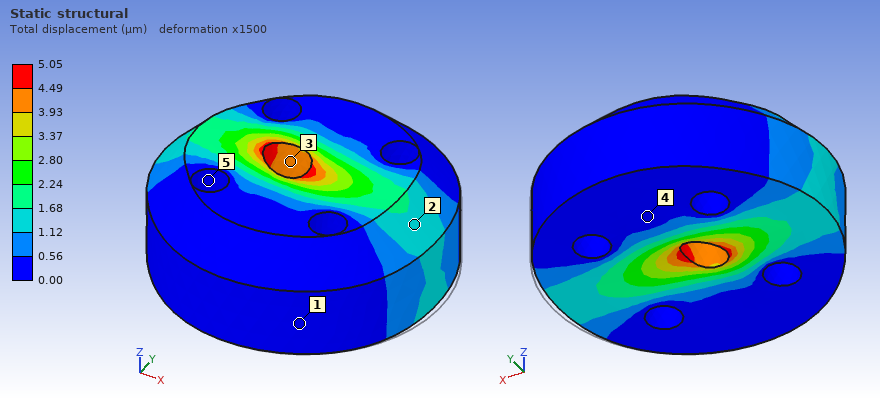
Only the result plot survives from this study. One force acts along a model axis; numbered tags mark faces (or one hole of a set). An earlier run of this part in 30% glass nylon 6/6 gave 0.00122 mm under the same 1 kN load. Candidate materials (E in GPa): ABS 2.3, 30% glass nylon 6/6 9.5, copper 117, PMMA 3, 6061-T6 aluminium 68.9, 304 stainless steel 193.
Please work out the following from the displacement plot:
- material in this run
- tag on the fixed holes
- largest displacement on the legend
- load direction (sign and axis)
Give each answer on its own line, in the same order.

ABS
5
5.05 µm
-X
